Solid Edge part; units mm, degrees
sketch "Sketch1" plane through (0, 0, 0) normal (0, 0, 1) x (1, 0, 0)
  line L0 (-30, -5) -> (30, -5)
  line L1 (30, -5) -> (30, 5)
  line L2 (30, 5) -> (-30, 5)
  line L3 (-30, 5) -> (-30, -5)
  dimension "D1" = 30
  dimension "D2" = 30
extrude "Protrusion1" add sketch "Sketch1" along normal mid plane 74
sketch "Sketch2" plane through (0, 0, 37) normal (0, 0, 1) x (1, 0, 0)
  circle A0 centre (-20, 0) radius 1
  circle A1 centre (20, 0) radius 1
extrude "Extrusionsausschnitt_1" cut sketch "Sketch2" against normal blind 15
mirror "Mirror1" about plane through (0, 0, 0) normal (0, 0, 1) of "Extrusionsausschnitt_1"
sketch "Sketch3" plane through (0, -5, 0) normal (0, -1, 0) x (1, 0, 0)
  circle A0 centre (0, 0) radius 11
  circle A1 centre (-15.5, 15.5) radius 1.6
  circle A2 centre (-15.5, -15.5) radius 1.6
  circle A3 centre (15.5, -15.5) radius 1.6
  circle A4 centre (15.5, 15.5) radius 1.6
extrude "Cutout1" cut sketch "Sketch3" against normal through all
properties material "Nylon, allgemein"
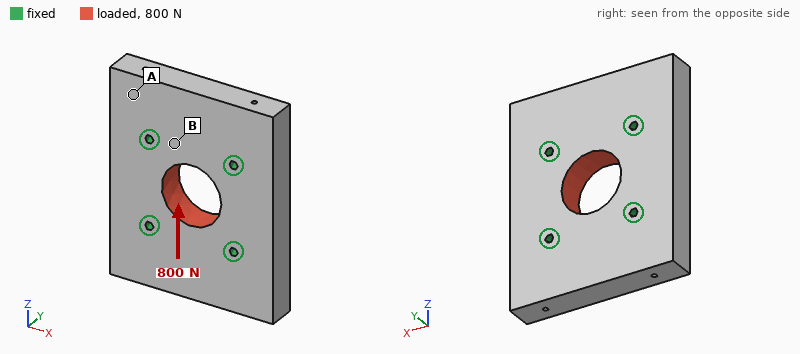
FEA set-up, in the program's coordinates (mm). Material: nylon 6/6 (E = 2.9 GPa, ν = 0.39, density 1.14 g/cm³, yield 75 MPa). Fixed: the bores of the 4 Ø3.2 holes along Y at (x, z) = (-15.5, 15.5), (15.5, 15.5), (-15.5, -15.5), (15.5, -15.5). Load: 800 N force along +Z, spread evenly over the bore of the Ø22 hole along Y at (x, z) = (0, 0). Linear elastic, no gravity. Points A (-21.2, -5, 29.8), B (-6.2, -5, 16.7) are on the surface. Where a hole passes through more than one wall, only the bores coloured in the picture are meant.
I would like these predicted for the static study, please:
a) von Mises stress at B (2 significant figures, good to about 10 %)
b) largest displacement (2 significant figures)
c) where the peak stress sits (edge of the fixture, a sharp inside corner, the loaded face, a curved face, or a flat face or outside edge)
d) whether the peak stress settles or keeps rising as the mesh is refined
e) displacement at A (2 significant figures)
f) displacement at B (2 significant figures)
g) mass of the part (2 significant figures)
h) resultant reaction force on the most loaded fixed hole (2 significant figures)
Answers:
0.89 MPa
10 µm
edge of the fixture
keeps rising
1.9 µm
6.7 µm
46 g
200 N
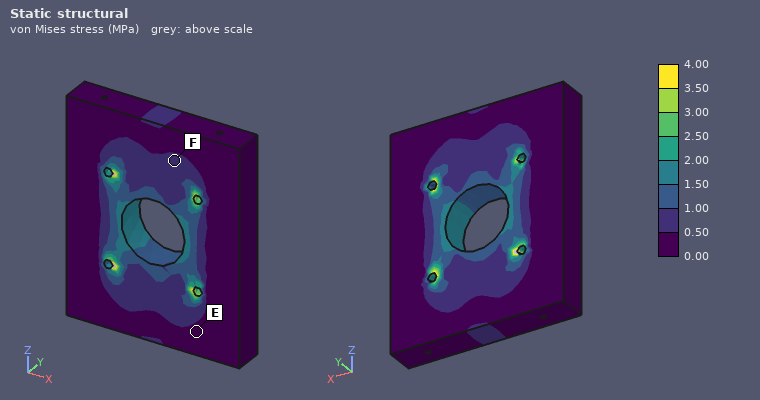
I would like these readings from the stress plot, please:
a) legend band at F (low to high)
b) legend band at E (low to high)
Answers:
0.50 to 1.00 MPa
0.00 to 0.50 MPa
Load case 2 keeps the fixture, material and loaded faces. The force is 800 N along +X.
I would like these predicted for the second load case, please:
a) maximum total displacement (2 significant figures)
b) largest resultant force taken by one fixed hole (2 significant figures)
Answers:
11 µm
200 N
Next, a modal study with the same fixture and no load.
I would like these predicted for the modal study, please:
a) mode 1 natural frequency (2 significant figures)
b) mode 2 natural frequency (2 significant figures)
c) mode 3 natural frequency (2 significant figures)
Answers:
3700 Hz
3800 Hz
4700 Hz
